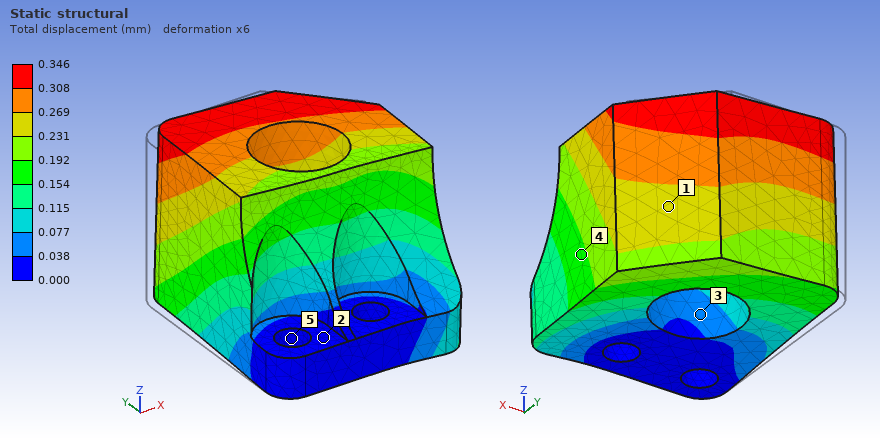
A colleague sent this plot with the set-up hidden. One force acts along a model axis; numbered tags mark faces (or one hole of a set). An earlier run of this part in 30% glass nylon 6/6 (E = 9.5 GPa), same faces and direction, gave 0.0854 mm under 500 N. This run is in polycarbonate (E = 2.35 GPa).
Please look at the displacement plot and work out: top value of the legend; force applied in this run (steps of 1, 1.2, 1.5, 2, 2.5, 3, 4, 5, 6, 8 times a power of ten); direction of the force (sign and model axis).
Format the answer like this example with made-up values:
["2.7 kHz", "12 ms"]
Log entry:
["0.346 mm", "500 N", "+X"]
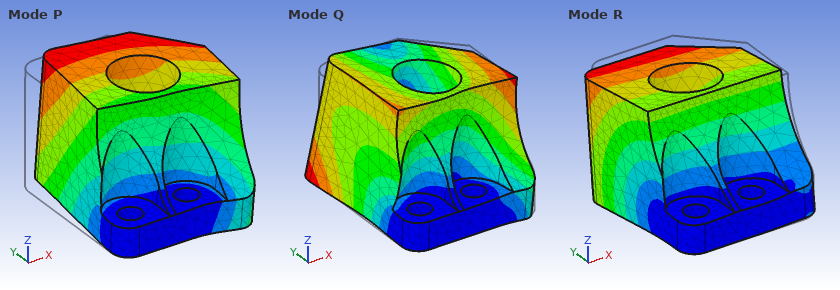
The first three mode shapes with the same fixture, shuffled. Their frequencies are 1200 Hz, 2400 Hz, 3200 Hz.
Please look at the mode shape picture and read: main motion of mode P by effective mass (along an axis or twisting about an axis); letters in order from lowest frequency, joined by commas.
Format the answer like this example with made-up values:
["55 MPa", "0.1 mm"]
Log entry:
["along X", "R, P, Q"]
